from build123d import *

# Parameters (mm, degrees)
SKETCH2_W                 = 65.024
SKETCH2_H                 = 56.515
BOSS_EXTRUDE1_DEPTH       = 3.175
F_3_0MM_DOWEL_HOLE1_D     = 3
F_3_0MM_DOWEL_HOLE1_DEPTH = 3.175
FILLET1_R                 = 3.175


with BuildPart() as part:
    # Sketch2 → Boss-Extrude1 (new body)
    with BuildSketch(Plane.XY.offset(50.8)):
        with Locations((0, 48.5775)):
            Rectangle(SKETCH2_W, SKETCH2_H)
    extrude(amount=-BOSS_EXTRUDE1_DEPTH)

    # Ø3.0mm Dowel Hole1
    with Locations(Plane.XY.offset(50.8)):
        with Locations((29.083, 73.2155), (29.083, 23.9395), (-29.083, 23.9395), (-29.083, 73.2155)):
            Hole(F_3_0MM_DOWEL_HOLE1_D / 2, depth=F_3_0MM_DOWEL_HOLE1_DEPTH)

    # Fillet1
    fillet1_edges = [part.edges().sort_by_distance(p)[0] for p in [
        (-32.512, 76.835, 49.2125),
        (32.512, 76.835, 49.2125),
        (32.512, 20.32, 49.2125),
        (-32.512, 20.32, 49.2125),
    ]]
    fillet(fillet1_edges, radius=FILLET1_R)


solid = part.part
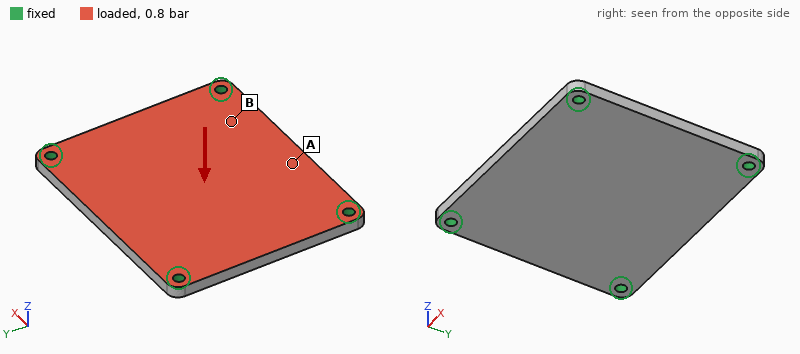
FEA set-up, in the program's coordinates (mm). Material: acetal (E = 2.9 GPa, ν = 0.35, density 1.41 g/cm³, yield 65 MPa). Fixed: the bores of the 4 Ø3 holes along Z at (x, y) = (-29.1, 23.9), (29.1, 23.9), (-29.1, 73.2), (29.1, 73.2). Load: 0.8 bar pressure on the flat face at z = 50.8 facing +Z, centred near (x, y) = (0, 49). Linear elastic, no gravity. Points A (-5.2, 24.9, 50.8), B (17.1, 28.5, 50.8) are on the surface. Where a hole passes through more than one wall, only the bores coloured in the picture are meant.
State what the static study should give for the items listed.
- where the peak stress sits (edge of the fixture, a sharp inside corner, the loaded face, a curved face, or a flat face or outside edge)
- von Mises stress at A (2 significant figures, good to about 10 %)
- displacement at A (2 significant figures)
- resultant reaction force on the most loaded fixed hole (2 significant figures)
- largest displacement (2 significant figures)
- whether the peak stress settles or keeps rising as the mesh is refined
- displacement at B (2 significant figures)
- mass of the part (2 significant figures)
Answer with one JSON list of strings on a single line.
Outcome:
["edge of the fixture", "8.5 MPa", "0.46 mm", "73 N", "0.66 mm", "keeps rising", "0.28 mm", "16 g"]
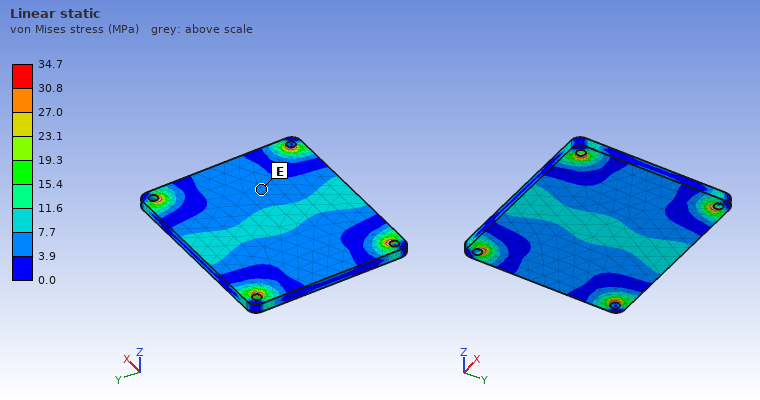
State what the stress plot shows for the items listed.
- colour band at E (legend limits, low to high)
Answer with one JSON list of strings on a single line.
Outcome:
["3.9 to 7.7 MPa"]
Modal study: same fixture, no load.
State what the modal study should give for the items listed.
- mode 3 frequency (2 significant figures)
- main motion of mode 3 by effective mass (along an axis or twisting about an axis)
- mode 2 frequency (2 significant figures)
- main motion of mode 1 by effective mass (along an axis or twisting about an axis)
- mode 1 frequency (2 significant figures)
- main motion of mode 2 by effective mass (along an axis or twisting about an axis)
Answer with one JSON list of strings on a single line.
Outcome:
["1900 Hz", "twisting about Y", "1600 Hz", "along Z", "990 Hz", "twisting about X"]
